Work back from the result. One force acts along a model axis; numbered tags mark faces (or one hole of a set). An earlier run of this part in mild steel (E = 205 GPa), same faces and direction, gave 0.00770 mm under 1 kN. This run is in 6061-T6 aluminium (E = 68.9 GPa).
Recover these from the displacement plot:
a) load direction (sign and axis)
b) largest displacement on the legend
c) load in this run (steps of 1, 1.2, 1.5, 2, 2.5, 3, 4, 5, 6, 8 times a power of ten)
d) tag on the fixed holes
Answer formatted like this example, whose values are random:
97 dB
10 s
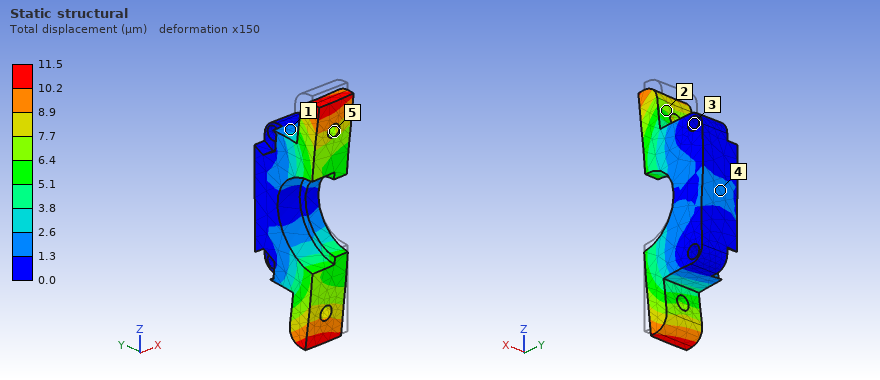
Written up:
-Z
11.5 µm
500 N
3
